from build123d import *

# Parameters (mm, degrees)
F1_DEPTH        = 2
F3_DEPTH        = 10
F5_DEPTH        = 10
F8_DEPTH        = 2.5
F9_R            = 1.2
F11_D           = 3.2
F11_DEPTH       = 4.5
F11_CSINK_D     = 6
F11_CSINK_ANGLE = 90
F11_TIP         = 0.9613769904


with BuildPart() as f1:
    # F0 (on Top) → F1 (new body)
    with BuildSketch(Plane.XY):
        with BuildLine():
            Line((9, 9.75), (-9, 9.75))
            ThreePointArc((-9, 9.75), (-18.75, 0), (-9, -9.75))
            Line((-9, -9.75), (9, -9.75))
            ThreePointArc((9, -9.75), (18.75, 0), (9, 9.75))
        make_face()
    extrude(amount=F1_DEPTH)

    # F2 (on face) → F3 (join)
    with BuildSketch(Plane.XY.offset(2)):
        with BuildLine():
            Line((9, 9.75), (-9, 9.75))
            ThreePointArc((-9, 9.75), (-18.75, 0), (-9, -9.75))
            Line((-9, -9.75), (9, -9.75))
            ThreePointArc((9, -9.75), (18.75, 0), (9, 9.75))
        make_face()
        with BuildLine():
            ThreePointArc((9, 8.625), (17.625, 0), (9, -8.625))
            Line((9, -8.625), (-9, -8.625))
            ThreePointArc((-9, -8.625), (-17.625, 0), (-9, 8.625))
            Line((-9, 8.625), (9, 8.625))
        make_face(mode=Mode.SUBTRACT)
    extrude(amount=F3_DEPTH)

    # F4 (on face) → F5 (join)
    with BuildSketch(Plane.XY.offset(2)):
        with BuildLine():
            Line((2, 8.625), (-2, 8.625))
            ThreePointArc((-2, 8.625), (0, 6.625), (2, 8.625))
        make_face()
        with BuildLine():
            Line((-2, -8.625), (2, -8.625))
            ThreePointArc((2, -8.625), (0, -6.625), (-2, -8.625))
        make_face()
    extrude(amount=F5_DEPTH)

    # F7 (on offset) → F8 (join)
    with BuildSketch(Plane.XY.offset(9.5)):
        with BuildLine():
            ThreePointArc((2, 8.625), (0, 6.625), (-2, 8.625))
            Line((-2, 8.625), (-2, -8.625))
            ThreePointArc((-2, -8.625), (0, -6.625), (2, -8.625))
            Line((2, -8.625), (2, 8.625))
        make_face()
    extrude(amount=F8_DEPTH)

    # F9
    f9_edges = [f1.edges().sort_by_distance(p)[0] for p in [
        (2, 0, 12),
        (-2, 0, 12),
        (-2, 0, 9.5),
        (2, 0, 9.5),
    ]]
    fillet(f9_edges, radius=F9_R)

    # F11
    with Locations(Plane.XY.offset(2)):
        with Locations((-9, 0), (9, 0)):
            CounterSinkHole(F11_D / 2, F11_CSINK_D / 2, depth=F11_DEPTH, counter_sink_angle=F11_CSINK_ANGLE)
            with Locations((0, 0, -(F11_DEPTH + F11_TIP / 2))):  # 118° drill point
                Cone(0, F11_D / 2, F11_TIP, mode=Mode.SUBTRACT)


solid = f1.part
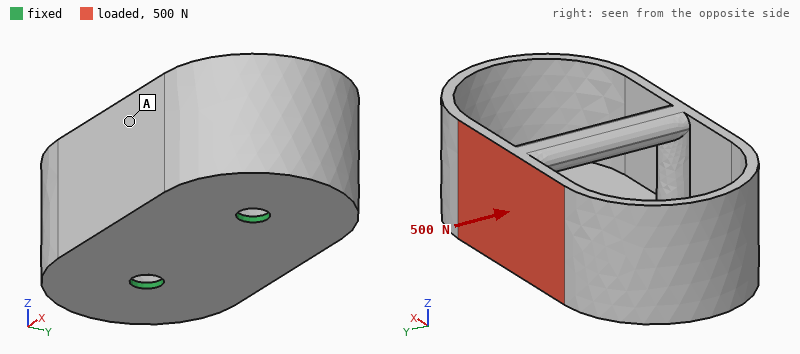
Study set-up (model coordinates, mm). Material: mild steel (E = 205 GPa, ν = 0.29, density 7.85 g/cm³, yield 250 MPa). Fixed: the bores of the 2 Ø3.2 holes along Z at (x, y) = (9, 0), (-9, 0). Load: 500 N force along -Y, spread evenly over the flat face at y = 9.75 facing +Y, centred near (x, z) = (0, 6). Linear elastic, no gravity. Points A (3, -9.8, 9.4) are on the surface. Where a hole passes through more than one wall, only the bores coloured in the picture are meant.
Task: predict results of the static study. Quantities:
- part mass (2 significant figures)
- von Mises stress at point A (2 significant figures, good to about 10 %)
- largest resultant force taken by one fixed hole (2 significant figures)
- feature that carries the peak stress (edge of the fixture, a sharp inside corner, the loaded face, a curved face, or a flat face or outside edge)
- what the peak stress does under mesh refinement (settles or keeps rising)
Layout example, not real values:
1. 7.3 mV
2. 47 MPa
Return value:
1. 20 g
2. 38 MPa
3. 250 N
4. edge of the fixture
5. keeps rising
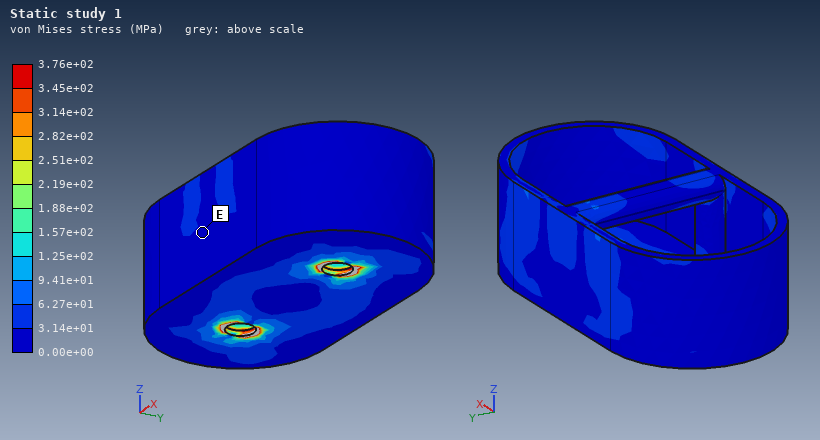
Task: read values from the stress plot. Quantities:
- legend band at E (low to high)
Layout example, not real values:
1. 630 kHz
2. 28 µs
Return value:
1. 0.00e+00 to 3.14e+01 MPa
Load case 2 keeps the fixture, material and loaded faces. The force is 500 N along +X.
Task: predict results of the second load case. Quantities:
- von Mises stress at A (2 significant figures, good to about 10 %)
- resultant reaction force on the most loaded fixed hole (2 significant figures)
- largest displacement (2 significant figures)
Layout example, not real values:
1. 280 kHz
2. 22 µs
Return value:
1. 19 MPa
2. 380 N
3. 15 µm
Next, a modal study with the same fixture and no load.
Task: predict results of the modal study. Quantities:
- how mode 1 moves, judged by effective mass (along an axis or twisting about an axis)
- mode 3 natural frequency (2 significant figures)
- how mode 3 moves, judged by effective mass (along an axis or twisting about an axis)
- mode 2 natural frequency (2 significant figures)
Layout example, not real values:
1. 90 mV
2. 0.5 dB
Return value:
1. along Y
2. 9100 Hz
3. along X
4. 8700 Hz
